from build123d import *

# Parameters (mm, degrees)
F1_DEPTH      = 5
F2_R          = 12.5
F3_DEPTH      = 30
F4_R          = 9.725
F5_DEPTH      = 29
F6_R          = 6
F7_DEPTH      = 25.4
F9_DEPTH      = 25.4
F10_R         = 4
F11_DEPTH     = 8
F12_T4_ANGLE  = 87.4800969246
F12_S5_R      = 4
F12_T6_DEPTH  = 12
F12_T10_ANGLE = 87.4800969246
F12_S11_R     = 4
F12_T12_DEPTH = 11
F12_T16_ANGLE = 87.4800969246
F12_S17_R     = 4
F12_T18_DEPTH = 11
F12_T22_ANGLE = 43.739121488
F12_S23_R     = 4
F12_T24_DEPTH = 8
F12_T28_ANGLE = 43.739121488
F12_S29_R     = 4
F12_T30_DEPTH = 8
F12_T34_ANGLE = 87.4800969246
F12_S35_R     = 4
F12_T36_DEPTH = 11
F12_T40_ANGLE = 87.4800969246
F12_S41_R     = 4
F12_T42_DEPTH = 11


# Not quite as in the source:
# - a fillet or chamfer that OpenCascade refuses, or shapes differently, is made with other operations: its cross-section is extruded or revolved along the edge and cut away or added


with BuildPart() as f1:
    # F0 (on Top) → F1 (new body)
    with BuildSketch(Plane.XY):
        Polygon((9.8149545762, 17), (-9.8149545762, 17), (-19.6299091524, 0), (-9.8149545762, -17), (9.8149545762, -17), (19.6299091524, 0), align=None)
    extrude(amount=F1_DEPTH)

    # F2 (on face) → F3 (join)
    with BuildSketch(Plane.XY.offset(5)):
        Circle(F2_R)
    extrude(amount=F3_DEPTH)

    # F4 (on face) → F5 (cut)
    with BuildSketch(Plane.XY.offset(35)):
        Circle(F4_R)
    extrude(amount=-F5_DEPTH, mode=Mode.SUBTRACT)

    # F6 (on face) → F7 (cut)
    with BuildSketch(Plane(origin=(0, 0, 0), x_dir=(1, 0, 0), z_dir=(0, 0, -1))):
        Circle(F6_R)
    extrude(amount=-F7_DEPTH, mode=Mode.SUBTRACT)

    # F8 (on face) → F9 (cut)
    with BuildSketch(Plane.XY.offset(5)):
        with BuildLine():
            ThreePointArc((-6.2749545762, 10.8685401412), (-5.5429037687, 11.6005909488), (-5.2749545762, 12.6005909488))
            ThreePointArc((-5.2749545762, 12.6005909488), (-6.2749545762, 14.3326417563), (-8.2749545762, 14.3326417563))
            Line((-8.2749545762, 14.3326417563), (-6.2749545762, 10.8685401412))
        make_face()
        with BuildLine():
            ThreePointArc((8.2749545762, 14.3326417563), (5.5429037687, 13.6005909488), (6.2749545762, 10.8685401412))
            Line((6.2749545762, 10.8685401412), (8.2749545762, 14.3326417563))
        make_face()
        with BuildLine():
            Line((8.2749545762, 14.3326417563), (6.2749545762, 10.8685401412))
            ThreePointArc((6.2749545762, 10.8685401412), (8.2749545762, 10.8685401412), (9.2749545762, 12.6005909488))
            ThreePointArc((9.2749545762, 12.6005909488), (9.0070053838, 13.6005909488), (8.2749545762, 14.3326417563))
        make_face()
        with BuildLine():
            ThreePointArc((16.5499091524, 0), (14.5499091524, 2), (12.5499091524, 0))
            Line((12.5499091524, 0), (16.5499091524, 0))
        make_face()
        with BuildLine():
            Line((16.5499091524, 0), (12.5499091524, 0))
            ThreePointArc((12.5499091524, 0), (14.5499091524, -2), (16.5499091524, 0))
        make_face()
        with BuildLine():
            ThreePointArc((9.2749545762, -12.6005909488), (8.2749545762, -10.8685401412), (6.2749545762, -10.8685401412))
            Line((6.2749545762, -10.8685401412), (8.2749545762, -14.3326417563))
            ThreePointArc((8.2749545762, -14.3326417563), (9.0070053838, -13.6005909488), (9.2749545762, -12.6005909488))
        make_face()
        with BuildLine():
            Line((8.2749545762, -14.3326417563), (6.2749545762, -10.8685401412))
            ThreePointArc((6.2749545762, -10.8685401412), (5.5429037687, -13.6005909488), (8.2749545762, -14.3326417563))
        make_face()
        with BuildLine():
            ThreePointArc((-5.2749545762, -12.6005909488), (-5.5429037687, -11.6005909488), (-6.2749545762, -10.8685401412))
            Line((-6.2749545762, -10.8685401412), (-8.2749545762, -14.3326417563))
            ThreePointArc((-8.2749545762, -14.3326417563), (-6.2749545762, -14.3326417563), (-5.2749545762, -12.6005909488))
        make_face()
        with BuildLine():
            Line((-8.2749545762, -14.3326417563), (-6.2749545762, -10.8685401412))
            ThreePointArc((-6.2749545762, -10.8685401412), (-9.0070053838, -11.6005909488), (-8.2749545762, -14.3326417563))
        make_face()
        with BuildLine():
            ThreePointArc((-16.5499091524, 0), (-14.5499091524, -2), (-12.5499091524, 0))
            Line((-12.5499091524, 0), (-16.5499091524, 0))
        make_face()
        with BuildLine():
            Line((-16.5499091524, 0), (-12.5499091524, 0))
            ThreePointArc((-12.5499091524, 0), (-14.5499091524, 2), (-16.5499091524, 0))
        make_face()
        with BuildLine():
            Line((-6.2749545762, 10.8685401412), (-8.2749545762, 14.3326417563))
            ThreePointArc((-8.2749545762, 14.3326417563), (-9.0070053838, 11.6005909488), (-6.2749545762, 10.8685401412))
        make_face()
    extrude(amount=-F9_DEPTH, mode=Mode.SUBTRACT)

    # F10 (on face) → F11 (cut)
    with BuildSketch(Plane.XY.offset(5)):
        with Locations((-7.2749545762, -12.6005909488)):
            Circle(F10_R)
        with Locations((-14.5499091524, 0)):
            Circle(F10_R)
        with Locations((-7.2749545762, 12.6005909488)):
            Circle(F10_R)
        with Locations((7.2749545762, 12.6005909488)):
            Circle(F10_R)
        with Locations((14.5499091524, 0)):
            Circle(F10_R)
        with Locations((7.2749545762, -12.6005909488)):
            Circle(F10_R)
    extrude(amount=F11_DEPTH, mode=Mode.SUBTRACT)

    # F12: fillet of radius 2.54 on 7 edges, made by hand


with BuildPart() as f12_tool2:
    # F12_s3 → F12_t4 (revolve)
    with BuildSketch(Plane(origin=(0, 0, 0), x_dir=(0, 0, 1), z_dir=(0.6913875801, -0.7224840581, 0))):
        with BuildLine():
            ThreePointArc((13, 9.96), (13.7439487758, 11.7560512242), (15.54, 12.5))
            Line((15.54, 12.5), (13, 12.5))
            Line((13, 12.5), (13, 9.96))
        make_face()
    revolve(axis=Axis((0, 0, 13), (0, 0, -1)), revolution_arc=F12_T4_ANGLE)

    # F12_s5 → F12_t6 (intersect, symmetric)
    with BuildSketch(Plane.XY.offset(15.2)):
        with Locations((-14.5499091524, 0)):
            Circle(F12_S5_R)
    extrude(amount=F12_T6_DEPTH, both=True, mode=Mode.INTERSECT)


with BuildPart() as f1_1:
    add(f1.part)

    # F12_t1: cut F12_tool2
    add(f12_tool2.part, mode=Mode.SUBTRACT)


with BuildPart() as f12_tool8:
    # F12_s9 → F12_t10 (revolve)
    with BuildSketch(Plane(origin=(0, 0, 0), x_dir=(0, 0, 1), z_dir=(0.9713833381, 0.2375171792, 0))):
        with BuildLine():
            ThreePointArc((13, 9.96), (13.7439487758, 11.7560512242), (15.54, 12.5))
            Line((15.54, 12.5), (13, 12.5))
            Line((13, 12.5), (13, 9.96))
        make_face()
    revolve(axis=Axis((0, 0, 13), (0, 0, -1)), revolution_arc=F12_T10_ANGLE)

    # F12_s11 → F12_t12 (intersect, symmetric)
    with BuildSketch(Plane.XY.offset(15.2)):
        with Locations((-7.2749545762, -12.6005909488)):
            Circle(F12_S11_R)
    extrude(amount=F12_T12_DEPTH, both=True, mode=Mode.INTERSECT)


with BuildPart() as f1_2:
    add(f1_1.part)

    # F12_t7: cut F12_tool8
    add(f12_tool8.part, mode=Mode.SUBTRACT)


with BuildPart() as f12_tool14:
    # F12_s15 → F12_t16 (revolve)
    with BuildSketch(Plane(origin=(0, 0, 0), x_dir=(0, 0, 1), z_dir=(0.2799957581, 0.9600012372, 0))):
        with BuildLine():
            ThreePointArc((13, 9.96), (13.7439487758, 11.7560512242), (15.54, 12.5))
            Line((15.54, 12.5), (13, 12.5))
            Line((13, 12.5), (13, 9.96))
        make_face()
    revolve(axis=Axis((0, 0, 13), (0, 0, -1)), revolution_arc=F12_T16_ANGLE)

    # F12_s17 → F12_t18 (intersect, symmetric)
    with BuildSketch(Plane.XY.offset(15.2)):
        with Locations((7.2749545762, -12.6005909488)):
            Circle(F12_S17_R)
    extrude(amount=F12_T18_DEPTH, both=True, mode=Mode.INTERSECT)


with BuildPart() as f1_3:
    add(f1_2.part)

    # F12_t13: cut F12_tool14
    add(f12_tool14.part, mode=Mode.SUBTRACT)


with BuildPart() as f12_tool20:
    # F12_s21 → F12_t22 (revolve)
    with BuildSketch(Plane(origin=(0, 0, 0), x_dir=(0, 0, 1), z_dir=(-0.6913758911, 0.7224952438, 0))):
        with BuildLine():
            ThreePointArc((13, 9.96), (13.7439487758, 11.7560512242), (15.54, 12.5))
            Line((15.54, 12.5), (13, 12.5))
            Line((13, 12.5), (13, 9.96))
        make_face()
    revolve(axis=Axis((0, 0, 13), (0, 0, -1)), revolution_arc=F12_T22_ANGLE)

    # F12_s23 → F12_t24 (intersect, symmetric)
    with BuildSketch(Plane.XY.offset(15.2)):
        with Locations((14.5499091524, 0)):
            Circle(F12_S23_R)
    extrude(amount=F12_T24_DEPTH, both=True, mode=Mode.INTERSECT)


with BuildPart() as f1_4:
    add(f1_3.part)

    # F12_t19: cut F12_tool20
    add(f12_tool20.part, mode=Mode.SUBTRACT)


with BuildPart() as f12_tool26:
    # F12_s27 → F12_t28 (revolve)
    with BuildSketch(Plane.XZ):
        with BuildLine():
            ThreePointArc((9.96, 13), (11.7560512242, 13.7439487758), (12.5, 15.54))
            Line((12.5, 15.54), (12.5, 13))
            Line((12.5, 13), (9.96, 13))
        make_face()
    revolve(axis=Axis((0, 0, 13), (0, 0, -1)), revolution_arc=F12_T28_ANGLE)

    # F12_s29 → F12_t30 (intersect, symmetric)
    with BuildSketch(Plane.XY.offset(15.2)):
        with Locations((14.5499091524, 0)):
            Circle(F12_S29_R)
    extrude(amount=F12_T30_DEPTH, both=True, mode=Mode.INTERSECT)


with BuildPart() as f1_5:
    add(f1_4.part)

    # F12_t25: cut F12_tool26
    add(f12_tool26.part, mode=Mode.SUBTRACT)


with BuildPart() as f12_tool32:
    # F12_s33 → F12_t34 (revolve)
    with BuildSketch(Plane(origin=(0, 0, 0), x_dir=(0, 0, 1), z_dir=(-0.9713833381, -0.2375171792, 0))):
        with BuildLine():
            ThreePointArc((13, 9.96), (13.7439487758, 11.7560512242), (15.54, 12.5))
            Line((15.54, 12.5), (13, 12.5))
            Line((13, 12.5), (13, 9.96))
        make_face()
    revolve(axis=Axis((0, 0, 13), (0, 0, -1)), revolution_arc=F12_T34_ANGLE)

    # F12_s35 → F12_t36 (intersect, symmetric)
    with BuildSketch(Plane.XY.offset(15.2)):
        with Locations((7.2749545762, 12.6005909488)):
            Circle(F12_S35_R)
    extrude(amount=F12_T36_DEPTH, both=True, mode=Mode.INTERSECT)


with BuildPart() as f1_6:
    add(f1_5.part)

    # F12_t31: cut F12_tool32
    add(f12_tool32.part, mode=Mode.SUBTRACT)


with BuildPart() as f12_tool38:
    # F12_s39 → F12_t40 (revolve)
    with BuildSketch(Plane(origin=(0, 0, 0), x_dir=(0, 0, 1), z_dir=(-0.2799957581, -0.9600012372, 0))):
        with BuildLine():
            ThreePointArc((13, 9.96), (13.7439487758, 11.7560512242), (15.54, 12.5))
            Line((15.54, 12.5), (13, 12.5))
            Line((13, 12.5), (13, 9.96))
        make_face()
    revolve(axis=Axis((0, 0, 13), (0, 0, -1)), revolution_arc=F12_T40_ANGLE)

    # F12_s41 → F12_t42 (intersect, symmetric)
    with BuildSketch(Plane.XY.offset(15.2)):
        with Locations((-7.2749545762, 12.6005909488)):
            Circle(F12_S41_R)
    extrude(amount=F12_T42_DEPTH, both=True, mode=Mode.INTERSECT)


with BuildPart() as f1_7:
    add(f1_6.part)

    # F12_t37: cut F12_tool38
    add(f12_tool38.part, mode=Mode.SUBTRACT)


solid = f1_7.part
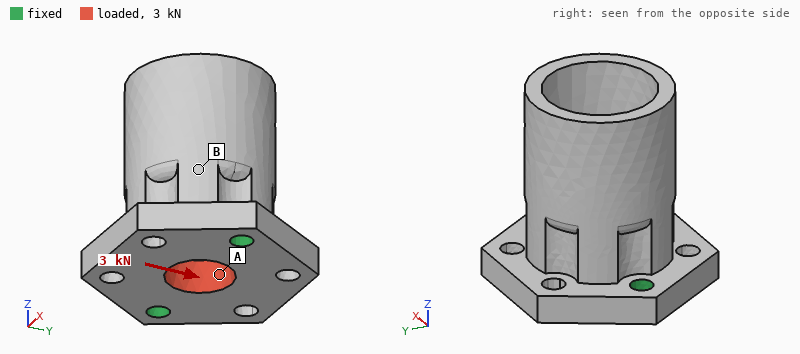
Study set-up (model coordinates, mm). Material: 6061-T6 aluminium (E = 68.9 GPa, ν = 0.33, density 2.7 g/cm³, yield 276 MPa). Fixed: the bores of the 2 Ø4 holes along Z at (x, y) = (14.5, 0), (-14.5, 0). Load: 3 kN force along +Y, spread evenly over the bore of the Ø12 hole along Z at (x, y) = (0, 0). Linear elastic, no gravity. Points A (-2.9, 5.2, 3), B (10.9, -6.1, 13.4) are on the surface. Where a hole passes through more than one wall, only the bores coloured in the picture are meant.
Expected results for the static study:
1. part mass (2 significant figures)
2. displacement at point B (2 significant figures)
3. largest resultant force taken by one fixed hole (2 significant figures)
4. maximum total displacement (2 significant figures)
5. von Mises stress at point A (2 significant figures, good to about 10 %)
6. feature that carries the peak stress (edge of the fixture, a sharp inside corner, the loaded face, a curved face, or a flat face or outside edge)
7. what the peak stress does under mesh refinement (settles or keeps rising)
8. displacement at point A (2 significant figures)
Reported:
26 g
6.1 µm
1.5 kN
11 µm
16 MPa
edge of the fixture
keeps rising
6.9 µm
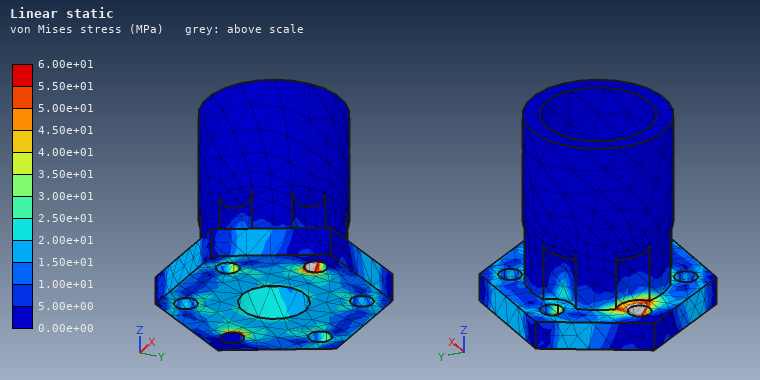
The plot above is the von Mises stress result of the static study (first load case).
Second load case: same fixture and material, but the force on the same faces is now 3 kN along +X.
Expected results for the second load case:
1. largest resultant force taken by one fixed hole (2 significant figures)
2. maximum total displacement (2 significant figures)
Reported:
1.5 kN
4.7 µm
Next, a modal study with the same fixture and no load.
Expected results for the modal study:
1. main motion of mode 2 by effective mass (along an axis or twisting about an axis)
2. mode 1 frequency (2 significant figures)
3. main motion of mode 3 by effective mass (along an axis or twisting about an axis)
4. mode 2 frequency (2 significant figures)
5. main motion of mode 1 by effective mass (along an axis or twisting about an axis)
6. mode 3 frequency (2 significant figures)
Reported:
along X
4400 Hz
along Z
10 kHz
along Y
14 kHz
